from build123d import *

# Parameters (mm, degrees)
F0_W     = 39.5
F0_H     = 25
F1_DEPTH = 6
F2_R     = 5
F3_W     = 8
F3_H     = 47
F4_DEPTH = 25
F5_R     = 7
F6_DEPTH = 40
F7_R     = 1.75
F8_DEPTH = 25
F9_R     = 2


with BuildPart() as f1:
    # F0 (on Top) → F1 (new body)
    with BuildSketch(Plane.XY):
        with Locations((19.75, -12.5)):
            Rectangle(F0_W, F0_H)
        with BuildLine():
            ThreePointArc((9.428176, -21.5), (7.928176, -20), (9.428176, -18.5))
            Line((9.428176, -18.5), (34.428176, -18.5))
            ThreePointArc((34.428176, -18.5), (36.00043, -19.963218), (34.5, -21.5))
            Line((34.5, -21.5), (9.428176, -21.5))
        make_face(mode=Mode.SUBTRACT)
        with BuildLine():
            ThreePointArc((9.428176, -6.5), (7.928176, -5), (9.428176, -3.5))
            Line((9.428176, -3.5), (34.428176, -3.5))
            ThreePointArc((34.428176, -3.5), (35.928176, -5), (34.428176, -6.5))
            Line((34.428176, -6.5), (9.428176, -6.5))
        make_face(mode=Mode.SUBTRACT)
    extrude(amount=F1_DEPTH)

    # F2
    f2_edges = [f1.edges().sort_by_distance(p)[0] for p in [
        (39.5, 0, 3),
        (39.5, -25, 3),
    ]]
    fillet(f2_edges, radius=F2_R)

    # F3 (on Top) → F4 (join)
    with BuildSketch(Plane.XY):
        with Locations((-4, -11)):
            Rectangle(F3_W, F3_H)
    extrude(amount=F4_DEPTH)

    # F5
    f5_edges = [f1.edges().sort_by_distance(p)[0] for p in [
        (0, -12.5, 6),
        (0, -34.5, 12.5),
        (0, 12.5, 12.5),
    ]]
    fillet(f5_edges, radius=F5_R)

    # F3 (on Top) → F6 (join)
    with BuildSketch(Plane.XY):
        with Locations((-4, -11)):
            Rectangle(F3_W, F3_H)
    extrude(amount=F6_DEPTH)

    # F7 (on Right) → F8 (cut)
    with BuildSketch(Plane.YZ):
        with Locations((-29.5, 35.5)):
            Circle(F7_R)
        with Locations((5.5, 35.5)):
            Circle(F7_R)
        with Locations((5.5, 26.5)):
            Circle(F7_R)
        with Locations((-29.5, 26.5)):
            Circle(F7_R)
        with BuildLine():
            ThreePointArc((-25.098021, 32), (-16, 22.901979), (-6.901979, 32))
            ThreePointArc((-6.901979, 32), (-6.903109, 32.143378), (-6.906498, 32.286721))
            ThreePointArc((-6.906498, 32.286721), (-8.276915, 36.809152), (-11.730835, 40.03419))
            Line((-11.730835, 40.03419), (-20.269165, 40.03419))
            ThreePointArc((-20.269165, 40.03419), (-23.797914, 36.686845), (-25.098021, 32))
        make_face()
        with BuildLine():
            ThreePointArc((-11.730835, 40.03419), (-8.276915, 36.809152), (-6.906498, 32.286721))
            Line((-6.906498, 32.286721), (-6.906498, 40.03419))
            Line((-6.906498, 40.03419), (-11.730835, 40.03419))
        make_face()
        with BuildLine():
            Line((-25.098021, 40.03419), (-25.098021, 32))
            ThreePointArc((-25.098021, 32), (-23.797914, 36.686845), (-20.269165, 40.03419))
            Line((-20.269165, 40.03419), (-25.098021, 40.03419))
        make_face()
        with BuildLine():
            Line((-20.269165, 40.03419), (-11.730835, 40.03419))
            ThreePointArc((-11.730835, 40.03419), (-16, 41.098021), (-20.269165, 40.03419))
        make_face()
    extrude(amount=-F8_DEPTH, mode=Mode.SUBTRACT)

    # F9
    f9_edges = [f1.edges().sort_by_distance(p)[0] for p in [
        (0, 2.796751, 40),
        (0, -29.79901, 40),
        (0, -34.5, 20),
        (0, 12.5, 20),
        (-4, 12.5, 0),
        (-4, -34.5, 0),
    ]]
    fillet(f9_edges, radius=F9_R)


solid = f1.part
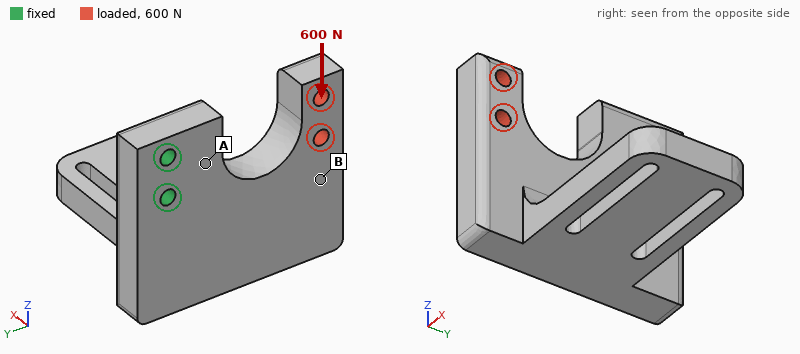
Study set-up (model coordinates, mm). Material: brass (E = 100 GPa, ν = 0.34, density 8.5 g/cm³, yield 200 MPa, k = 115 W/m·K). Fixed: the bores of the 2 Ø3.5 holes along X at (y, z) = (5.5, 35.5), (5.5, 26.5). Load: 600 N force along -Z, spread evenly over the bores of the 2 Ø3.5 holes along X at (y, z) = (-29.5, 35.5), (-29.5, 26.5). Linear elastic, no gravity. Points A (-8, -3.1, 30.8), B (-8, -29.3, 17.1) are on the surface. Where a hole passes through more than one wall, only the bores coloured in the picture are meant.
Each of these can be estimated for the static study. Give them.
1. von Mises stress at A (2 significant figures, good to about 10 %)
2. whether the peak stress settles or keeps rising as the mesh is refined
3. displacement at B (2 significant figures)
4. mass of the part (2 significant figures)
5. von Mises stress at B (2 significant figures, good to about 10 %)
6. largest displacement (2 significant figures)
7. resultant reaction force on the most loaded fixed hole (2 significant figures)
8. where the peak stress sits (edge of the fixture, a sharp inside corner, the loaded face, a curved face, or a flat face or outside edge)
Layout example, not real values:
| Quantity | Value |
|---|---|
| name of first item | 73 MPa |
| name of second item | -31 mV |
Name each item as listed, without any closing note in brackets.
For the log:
| Quantity | Value |
|---|---|
| von Mises stress at A | 28 MPa |
| whether the peak stress settles or keeps rising as the mesh is refined | keeps rising |
| displacement at B | 30 µm |
| mass of the part | 150 g |
| von Mises stress at B | 6.2 MPa |
| largest displacement | 40 µm |
| resultant reaction force on the most loaded fixed hole | 1.7 kN |
| where the peak stress sits | edge of the fixture |
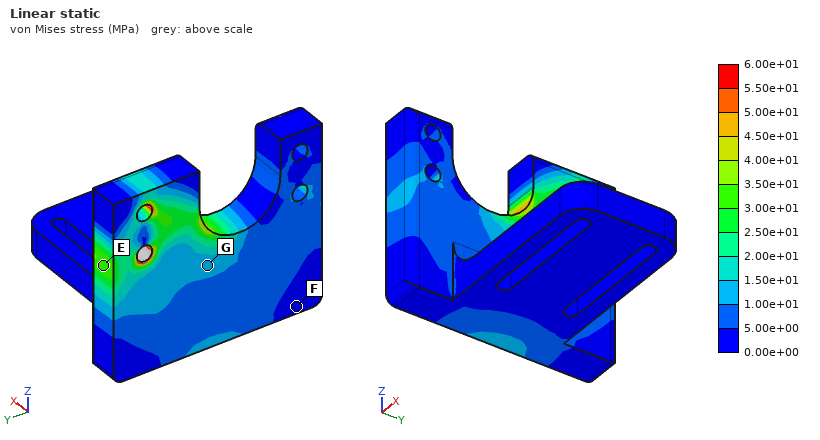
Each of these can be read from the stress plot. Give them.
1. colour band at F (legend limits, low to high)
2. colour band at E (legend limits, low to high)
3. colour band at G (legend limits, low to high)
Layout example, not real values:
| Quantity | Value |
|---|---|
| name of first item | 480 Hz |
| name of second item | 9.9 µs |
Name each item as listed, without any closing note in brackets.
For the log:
| Quantity | Value |
|---|---|
| colour band at F | 0.00e+00 to 5.00e+00 MPa |
| colour band at E | 3.00e+01 to 3.50e+01 MPa |
| colour band at G | 1.00e+01 to 1.50e+01 MPa |
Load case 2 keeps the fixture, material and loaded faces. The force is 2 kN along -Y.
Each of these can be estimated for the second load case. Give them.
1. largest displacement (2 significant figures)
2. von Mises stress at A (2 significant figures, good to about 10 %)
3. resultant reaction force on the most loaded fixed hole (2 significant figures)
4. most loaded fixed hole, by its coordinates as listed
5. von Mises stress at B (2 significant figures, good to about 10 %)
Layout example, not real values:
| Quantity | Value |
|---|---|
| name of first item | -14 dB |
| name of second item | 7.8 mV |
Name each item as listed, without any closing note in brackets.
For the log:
| Quantity | Value |
|---|---|
| largest displacement | 81 µm |
| von Mises stress at A | 18 MPa |
| resultant reaction force on the most loaded fixed hole | 1.2 kN |
| most loaded fixed hole, by its coordinates as listed | (5.5, 26.5) |
| von Mises stress at B | 23 MPa |
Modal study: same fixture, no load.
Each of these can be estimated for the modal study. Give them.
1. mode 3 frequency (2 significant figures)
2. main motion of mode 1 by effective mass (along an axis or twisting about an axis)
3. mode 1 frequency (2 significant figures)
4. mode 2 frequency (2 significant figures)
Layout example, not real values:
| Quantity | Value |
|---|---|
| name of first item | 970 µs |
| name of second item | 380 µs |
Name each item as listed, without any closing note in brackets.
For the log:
| Quantity | Value |
|---|---|
| mode 3 frequency | 2800 Hz |
| main motion of mode 1 by effective mass | along X |
| mode 1 frequency | 1200 Hz |
| mode 2 frequency | 1500 Hz |
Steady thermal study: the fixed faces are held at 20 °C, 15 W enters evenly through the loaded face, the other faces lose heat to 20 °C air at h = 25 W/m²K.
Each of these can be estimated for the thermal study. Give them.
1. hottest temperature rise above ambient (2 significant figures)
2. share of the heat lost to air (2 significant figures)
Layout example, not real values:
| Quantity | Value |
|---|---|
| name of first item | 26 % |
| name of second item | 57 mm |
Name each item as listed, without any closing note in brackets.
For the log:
| Quantity | Value |
|---|---|
| hottest temperature rise above ambient | 44 K |
| share of the heat lost to air | 17 % |
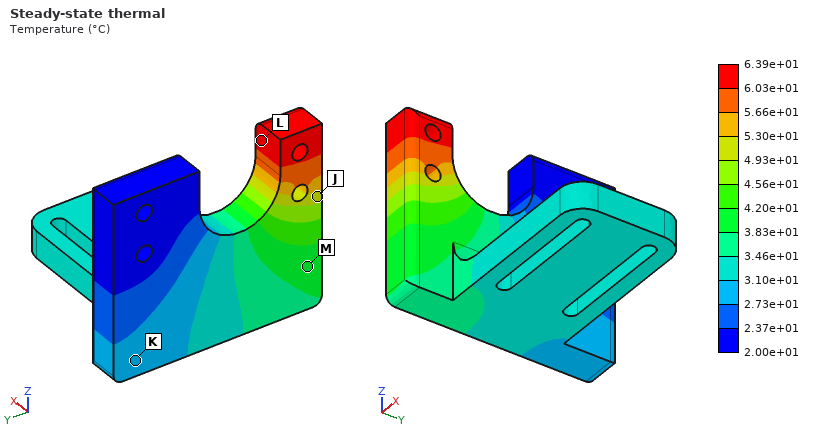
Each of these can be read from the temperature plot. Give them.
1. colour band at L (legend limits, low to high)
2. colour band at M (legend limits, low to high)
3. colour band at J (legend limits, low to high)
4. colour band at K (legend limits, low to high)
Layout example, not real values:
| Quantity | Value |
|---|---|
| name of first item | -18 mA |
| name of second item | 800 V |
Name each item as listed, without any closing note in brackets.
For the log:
| Quantity | Value |
|---|---|
| colour band at L | 6.03e+01 to 6.39e+01 °C |
| colour band at M | 3.83e+01 to 4.20e+01 °C |
| colour band at J | 4.93e+01 to 5.30e+01 °C |
| colour band at K | 2.73e+01 to 3.10e+01 °C |
